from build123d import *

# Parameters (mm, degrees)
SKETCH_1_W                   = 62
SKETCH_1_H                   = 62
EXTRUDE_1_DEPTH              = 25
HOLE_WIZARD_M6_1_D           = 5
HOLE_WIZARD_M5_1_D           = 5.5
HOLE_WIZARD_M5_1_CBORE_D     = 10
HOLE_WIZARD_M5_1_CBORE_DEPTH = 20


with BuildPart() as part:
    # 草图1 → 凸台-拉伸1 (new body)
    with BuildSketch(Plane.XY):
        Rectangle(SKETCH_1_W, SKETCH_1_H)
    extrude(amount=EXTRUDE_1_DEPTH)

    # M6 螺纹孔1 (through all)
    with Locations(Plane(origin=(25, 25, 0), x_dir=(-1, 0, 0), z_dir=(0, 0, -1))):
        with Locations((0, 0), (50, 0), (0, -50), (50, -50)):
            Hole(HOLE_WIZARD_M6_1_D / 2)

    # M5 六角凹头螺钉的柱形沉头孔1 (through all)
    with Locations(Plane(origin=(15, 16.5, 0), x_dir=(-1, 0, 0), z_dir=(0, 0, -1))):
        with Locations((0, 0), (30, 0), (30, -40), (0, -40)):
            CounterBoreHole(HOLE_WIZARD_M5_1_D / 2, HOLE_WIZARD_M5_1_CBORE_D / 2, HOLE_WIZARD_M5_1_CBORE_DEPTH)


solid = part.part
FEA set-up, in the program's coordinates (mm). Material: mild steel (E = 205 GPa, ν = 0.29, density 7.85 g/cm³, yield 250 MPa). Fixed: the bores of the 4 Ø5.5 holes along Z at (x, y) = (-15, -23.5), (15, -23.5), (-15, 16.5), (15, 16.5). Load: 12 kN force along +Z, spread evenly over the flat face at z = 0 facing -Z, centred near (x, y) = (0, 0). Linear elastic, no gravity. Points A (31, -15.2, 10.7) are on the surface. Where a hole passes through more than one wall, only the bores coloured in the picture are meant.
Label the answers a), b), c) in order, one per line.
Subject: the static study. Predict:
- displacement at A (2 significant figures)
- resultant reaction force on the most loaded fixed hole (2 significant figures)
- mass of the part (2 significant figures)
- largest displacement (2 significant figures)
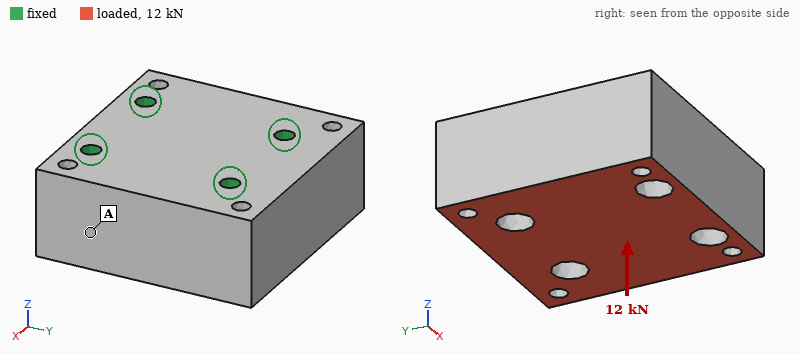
a) 2.3 µm
b) 3.6 kN
c) 690 g
d) 2.8 µm
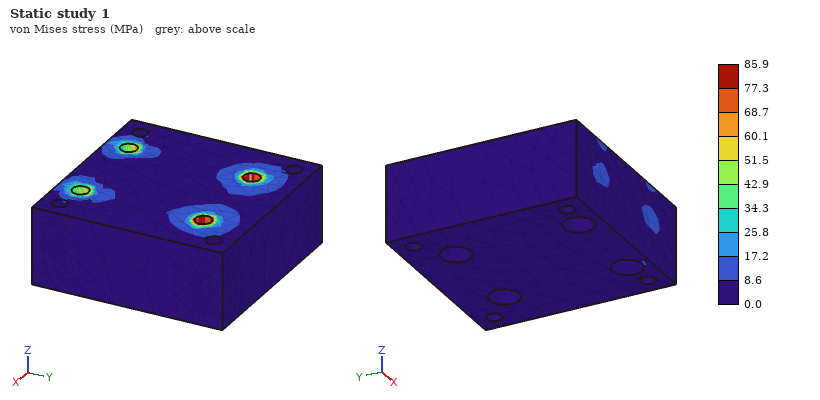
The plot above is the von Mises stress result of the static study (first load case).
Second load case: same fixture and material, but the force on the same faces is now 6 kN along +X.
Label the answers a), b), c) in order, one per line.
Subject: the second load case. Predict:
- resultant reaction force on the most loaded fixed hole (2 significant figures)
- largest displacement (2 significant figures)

a) 2.8 kN
b) 5.2 µm
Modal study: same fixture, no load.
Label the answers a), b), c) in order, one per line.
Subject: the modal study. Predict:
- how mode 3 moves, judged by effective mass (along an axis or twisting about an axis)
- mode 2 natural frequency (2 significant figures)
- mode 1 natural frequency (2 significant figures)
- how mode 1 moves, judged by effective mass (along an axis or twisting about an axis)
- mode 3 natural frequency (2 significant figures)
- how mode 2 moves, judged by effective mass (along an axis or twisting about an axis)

a) along Z
b) 13 kHz
c) 9900 Hz
d) along X
e) 15 kHz
f) along Y
